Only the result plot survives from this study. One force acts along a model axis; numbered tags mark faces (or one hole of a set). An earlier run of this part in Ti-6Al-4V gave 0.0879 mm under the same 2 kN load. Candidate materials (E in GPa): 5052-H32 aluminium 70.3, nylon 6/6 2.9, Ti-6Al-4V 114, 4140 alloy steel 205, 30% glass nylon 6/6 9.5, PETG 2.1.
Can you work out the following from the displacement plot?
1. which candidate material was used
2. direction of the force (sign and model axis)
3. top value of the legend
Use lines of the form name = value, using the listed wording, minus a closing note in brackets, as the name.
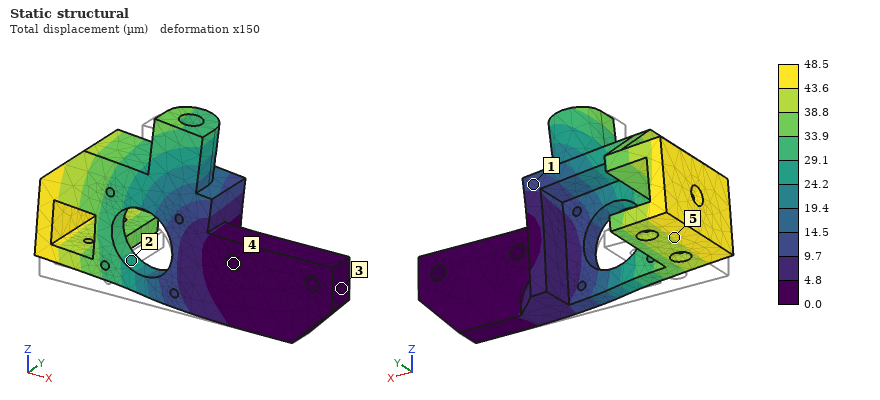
which candidate material was used = 4140 alloy steel
direction of the force = +Z
top value of the legend = 48.5 µm
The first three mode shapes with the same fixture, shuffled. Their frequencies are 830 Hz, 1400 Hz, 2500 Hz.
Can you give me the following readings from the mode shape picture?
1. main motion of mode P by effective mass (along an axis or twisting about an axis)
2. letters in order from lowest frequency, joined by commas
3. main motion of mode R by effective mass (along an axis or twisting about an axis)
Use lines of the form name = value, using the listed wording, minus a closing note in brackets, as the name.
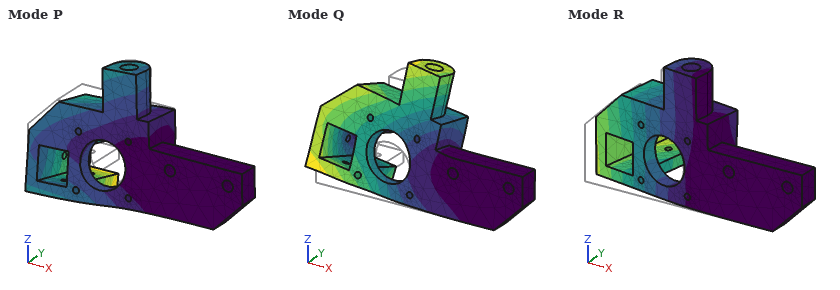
main motion of mode P by effective mass = along Z
letters in order from lowest frequency, joined by commas = R, P, Q
main motion of mode R by effective mass = along Y
